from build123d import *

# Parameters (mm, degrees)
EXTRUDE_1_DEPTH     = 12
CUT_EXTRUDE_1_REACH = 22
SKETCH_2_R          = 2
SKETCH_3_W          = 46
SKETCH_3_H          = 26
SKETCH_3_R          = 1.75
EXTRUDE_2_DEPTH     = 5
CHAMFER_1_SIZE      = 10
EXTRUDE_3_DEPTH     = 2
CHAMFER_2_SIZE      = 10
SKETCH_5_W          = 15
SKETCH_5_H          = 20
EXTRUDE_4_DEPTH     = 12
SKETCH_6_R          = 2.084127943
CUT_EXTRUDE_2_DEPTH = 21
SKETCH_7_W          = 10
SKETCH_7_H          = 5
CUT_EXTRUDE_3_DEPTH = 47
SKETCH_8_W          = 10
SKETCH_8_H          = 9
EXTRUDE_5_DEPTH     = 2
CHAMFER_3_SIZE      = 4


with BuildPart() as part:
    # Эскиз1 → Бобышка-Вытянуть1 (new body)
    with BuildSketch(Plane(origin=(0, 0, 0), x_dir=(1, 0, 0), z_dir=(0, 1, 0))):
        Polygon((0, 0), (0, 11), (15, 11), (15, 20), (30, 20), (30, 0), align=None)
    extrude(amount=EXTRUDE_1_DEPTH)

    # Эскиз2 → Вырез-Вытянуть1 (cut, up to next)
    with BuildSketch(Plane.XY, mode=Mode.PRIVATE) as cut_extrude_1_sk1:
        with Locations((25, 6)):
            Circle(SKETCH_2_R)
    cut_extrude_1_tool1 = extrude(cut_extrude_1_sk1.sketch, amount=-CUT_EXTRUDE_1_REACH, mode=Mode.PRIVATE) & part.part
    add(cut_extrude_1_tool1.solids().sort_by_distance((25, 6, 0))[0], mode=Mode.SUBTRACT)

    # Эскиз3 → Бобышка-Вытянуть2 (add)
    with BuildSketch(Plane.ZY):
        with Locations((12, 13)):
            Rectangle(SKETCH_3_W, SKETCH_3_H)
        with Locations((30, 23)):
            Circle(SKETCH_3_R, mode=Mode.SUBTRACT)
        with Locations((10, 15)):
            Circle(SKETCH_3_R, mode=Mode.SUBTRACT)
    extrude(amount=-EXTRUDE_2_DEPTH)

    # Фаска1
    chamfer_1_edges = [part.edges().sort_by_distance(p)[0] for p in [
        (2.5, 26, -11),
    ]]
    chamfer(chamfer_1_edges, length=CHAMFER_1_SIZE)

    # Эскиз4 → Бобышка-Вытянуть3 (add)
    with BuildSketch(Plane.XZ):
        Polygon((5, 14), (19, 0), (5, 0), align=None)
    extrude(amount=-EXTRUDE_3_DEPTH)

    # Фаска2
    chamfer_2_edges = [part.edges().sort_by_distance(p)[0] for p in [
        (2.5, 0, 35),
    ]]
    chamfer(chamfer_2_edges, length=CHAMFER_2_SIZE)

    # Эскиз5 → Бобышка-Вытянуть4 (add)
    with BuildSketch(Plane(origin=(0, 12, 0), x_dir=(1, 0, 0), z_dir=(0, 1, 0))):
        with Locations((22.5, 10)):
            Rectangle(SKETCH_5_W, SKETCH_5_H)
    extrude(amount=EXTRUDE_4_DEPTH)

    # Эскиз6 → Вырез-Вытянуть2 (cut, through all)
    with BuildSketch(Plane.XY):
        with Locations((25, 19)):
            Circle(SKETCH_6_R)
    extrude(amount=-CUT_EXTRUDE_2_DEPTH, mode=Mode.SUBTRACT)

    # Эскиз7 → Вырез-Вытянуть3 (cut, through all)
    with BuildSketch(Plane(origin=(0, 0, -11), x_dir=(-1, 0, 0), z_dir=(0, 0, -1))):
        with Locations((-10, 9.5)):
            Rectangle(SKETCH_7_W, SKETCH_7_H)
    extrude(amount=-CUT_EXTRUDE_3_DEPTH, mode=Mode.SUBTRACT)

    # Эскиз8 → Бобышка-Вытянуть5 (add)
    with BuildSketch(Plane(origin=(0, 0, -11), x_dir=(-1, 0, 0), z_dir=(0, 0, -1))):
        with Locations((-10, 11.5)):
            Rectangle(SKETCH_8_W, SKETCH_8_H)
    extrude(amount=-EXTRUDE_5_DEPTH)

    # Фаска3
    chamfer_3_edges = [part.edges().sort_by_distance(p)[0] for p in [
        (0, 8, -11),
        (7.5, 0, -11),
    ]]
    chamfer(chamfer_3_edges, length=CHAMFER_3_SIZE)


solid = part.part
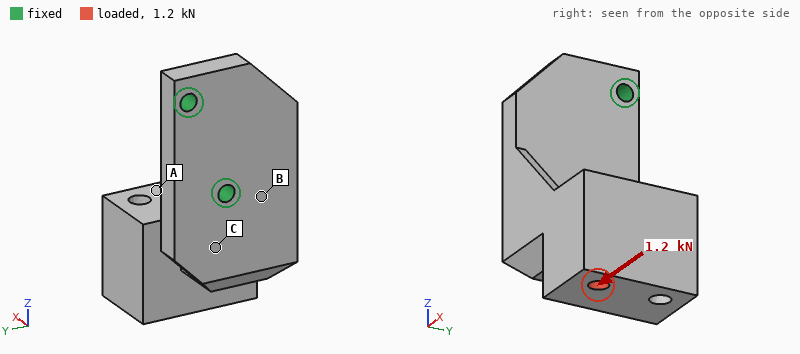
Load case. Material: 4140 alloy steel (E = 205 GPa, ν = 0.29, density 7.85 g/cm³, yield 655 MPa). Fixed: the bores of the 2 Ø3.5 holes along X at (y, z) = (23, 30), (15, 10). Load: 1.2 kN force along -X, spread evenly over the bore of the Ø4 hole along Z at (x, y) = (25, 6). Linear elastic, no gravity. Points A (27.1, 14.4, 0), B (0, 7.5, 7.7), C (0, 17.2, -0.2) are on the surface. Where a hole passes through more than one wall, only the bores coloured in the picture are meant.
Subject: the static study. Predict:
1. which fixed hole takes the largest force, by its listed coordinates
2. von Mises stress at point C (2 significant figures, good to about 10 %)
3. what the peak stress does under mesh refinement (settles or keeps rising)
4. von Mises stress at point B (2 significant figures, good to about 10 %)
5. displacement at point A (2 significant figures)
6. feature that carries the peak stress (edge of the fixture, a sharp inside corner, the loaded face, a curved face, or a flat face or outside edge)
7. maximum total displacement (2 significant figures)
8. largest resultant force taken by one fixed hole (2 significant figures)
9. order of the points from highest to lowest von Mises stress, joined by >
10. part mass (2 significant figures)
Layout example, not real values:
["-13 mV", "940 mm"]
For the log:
["(15, 10)", "110 MPa", "keeps rising", "160 MPa", "0.13 mm", "edge of the fixture", "0.21 mm", "1.7 kN", "B > C > A", "100 g"]
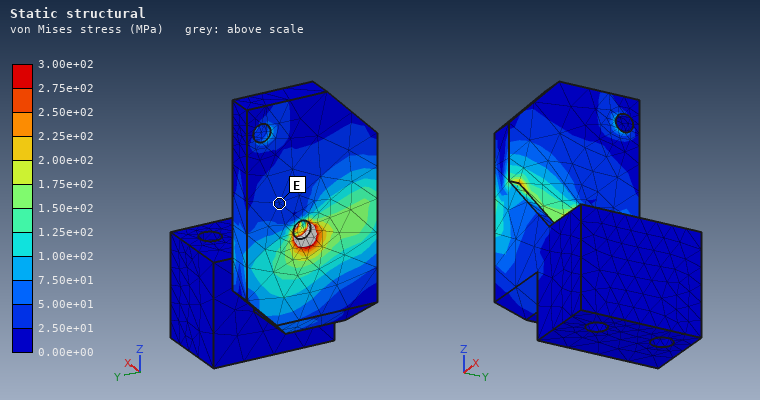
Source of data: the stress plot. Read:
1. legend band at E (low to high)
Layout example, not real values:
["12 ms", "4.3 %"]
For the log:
["2.50e+01 to 5.00e+01 MPa"]
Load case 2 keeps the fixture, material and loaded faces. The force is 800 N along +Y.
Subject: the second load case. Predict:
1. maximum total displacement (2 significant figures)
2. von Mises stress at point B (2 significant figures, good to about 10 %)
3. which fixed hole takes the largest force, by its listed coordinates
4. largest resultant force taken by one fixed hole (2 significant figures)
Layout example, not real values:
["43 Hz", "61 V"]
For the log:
["0.21 mm", "120 MPa", "(15, 10)", "1.4 kN"]
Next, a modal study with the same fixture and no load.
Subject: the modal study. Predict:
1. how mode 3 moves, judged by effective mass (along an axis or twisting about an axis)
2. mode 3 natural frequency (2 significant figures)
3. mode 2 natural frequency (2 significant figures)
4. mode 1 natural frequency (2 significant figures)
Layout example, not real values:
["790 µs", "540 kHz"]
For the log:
["along X", "4400 Hz", "2000 Hz", "1500 Hz"]
